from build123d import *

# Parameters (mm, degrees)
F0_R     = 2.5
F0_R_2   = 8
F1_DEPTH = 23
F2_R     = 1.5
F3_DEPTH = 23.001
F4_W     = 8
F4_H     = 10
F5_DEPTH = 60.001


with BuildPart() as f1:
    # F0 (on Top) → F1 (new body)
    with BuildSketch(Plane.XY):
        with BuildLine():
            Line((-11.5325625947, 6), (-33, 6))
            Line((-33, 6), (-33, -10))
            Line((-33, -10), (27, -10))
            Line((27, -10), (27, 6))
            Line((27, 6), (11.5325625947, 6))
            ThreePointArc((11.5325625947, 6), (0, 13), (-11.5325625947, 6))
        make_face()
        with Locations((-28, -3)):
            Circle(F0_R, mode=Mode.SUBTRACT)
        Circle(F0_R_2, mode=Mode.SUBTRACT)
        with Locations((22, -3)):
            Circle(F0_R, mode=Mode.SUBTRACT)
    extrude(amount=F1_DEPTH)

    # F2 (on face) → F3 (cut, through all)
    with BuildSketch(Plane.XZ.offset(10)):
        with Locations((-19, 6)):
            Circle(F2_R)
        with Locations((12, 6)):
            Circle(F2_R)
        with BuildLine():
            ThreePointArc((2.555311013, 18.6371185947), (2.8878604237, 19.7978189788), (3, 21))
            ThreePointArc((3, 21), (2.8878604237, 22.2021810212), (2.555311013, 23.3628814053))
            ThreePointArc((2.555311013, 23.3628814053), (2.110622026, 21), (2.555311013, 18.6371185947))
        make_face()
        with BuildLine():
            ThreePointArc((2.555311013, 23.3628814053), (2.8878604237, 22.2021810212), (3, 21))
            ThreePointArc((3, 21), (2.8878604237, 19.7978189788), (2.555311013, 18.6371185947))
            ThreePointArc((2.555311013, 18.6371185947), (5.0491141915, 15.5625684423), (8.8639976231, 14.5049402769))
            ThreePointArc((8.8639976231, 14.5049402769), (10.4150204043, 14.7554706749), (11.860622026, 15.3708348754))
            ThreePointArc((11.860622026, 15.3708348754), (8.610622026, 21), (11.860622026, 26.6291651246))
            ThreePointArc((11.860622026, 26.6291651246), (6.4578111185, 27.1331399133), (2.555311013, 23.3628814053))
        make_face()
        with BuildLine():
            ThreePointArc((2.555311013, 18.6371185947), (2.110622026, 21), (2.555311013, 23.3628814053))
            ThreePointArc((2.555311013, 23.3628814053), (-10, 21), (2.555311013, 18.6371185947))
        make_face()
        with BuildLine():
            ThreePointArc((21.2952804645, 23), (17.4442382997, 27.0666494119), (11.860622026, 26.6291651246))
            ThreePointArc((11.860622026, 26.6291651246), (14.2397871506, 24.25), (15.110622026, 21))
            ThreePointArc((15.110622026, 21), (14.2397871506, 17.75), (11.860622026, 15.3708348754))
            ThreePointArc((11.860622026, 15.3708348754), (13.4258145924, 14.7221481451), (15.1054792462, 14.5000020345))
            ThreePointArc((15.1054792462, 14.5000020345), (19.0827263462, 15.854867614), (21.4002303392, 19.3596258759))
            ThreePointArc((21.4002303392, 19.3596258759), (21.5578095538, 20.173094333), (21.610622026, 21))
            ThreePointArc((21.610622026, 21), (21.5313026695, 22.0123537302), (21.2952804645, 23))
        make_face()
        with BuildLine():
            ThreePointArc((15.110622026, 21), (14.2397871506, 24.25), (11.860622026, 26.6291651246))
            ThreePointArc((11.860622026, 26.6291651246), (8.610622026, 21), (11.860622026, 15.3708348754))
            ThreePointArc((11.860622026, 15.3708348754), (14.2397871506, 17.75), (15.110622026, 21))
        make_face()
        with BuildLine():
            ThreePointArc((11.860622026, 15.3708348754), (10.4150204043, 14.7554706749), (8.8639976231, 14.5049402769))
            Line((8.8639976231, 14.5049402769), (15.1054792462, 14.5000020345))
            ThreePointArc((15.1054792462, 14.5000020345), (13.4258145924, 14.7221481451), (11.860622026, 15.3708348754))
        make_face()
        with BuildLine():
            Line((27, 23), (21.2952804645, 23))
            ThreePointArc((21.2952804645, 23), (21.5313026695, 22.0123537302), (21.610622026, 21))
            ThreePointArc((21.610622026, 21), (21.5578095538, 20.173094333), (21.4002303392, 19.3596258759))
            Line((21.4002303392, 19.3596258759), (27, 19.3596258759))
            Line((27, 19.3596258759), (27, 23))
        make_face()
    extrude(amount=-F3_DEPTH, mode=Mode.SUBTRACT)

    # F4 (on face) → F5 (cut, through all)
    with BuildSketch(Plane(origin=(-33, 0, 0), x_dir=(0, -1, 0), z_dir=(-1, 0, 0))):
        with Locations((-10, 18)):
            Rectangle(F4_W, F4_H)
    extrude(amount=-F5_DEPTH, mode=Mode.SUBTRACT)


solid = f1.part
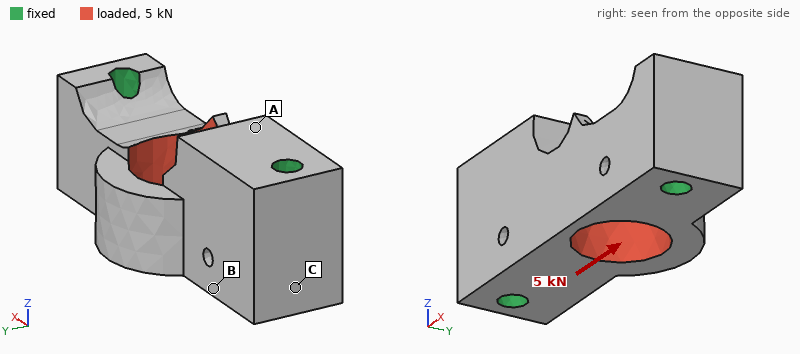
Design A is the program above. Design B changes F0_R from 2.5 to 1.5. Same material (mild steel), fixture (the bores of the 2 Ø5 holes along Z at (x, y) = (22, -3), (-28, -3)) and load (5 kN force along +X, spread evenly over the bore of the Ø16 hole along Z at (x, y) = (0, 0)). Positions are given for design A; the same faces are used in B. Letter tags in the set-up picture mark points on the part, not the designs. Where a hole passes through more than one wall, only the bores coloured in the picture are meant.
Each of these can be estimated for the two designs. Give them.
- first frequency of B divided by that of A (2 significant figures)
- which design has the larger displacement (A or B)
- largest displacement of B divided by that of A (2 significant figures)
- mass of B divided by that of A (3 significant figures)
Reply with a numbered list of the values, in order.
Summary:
1. 0.79
2. B
3. 1.1
4. 1.03
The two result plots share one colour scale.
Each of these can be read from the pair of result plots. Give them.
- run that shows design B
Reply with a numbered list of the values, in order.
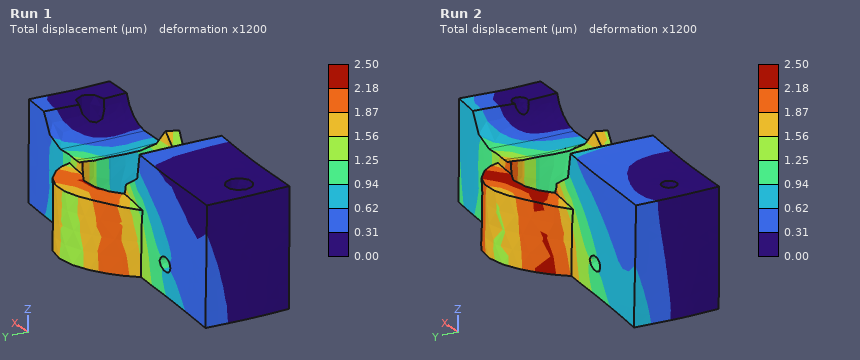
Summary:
1. Run 2
